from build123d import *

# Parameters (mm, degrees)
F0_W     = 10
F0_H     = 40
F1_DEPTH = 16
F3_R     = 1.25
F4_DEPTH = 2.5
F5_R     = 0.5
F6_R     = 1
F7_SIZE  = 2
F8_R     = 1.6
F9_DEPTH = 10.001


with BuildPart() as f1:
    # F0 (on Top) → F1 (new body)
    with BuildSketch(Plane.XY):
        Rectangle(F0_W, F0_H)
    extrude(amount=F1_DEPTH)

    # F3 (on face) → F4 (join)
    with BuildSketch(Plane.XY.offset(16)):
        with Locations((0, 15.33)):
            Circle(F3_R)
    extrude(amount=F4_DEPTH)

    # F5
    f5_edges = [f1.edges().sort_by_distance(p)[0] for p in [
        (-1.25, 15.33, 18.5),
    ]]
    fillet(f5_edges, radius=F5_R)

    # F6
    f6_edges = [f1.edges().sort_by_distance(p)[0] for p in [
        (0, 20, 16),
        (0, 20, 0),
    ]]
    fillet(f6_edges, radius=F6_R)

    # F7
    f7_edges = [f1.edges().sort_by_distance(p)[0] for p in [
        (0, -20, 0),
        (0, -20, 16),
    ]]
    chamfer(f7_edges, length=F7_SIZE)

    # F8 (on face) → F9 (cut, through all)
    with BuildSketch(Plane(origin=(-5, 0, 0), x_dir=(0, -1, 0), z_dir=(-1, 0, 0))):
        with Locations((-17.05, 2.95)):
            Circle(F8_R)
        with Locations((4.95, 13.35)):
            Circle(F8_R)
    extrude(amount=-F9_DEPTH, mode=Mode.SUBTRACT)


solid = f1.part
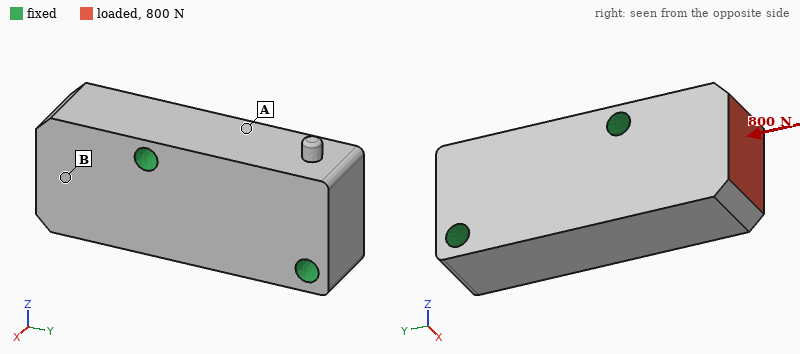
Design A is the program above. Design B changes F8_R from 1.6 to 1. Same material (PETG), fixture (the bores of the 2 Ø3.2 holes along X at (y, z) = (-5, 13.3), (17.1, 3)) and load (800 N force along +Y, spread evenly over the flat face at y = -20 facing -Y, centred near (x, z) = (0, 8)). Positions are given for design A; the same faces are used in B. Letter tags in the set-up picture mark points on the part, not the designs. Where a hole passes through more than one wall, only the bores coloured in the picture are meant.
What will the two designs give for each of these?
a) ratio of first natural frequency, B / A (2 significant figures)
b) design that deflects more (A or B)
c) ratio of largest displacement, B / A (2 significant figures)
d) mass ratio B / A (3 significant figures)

0.88
B
1.1
1.02
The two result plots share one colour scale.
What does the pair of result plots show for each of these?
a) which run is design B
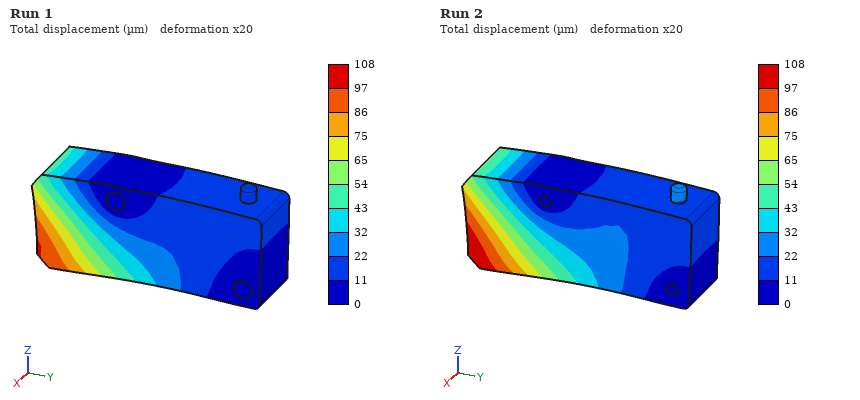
Run 2
